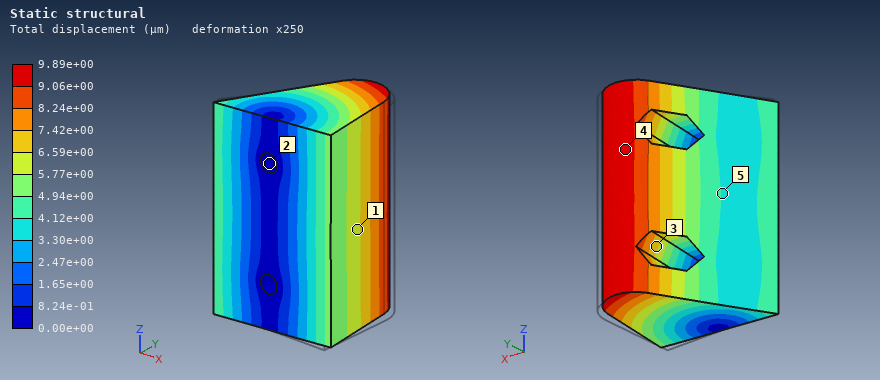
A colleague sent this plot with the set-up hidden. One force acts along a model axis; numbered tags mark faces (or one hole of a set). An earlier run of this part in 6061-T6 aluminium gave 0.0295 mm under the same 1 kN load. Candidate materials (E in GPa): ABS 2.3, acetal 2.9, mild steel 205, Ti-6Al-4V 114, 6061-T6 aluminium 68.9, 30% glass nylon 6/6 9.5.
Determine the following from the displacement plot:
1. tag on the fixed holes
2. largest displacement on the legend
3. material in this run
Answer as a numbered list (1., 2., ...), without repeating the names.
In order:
1. 2
2. 9.89e+00 µm
3. mild steel
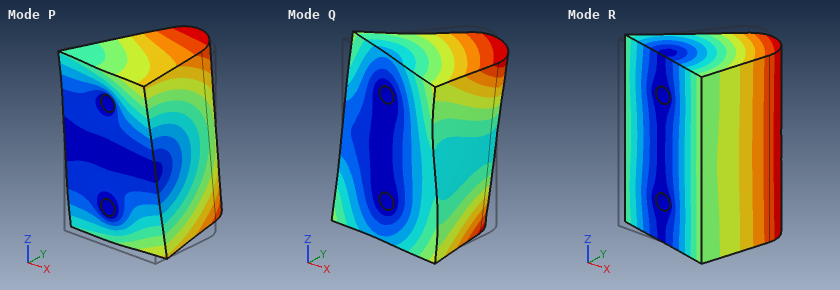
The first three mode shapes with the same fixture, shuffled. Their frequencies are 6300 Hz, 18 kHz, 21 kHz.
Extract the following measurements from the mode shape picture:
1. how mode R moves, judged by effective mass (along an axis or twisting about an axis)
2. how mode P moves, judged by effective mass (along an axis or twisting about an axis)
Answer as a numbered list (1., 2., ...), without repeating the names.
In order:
1. along X
2. along Z
